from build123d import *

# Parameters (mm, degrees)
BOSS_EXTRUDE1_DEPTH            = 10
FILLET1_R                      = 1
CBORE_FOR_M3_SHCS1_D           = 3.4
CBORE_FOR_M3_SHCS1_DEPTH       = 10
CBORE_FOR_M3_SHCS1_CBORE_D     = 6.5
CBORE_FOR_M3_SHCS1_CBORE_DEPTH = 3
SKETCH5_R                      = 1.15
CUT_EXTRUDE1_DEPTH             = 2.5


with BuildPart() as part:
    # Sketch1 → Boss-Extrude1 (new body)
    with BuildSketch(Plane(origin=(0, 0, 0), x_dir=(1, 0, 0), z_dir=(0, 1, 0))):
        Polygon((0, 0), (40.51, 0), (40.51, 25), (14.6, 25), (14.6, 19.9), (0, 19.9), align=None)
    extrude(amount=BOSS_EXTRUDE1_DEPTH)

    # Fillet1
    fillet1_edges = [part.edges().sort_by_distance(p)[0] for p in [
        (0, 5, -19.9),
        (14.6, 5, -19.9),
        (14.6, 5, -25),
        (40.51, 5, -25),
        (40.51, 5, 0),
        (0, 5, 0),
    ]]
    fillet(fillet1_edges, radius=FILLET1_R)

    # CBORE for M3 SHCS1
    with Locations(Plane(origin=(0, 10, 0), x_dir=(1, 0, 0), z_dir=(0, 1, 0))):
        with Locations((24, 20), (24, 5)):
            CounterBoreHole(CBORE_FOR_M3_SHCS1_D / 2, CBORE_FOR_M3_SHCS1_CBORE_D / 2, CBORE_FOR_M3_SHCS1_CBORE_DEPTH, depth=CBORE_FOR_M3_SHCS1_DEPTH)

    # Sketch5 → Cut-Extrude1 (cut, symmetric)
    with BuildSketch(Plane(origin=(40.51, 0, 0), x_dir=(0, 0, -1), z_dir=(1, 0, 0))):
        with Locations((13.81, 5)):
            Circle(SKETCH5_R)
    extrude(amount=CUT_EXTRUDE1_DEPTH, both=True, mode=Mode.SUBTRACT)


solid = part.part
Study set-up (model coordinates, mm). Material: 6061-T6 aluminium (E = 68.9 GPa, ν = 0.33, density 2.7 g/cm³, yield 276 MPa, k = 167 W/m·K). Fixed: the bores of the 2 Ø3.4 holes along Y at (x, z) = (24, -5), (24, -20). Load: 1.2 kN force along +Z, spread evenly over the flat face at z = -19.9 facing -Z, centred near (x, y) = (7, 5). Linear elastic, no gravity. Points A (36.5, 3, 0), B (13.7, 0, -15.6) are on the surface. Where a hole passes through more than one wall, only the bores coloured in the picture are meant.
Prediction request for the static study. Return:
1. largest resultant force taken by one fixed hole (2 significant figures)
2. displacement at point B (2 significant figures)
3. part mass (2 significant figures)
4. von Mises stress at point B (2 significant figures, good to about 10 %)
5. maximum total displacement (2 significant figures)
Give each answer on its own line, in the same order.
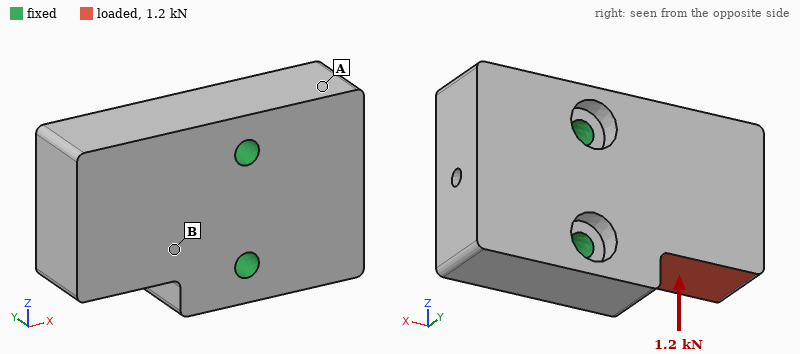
1.3 kN
4.0 µm
24 g
17 MPa
11 µm
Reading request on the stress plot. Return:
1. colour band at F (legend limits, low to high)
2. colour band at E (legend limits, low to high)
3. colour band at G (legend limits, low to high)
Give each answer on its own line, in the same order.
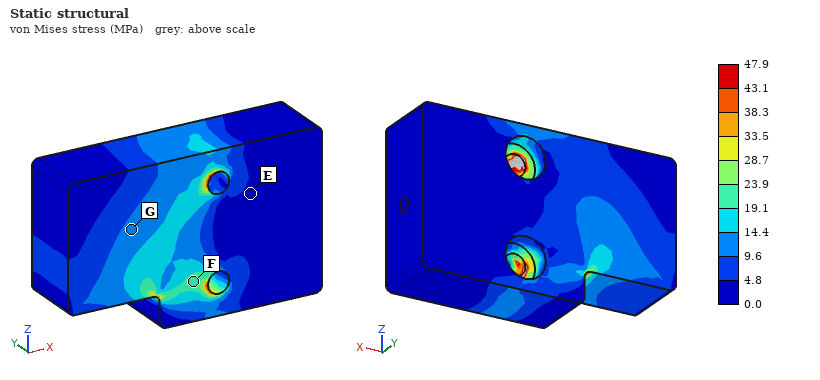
19.1 to 23.9 MPa
0.0 to 4.8 MPa
9.6 to 14.4 MPa
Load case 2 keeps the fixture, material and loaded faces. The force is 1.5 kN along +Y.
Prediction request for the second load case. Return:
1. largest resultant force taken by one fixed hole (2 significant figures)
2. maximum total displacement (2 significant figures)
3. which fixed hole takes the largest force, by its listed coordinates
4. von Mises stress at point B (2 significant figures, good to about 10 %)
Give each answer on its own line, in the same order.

1.4 kN
75 µm
(24, -20)
59 MPa
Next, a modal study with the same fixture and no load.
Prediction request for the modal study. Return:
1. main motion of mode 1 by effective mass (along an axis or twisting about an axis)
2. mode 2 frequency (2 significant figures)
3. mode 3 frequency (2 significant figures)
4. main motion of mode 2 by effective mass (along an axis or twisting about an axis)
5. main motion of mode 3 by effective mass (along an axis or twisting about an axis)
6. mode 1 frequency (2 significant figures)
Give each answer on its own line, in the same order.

along Y
19 kHz
21 kHz
along Y
along Z
10000 Hz
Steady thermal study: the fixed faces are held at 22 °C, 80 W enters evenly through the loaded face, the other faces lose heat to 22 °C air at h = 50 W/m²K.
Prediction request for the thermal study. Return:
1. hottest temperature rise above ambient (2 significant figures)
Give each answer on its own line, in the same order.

58 K
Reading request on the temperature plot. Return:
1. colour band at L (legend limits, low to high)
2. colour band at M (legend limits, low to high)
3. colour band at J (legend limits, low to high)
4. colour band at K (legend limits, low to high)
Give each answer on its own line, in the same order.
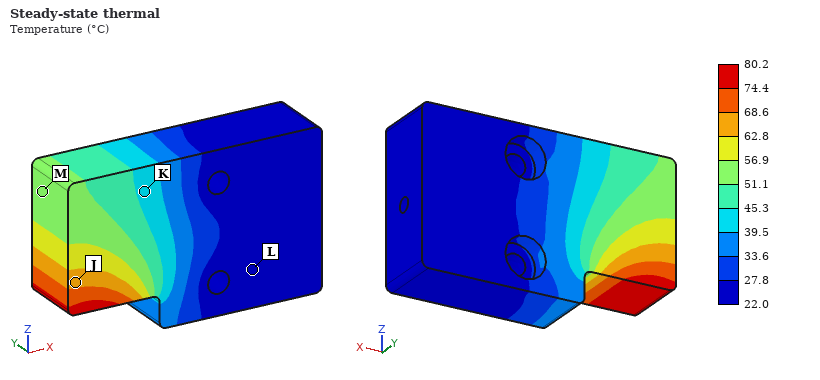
22.0 to 27.8 °C
51.1 to 56.9 °C
62.8 to 68.6 °C
39.5 to 45.3 °C
